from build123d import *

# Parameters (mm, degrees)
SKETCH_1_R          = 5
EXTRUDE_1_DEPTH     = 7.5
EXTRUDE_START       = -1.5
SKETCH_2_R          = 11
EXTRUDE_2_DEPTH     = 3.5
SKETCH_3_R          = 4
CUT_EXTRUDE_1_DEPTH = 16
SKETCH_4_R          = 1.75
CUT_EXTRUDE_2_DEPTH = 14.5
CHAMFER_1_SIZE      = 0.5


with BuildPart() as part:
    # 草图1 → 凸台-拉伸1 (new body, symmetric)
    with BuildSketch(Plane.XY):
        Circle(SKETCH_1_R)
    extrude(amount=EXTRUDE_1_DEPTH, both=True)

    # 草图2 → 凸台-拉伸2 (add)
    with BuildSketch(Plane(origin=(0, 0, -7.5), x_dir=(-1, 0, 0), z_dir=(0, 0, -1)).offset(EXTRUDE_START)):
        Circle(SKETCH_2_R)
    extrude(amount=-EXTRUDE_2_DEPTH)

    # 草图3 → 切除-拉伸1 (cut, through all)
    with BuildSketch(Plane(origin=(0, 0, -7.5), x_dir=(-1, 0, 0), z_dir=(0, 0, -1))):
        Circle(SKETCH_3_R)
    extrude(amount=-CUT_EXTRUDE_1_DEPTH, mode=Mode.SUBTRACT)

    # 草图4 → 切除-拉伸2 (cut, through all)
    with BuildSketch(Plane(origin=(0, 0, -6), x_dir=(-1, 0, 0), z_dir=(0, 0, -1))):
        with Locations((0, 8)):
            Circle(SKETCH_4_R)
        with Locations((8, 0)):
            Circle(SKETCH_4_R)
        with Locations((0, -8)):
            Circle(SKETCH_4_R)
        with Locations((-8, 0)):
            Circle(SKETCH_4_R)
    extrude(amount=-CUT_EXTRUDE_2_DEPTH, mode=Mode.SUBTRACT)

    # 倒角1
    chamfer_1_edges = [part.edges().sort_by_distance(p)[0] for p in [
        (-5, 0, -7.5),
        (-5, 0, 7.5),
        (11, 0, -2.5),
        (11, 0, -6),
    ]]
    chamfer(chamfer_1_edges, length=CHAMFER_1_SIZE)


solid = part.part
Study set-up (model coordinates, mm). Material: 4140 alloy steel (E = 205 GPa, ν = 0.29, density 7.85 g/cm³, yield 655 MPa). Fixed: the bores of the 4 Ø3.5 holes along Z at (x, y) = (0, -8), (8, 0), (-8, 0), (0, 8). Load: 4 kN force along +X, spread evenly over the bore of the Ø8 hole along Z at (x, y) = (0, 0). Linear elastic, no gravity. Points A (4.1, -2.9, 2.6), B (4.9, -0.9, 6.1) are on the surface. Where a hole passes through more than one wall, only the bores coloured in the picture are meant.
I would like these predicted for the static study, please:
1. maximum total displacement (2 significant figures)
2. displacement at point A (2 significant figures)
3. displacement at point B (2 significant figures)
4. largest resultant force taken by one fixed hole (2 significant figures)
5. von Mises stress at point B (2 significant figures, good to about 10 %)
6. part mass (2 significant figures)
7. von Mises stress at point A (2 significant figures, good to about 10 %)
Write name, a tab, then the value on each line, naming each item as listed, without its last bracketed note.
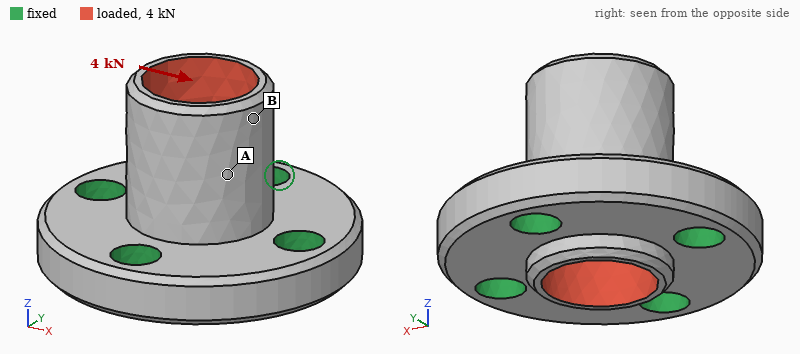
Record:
maximum total displacement	26 µm
displacement at point A	16 µm
displacement at point B	23 µm
largest resultant force taken by one fixed hole	1.7 kN
von Mises stress at point B	50 MPa
part mass	10 g
von Mises stress at point A	100 MPa
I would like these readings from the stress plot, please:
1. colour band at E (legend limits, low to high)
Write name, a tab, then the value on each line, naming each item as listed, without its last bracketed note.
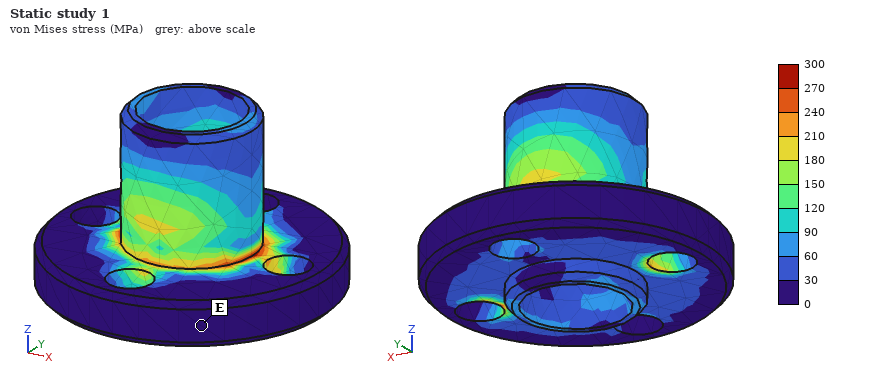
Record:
colour band at E	0 to 30 MPa
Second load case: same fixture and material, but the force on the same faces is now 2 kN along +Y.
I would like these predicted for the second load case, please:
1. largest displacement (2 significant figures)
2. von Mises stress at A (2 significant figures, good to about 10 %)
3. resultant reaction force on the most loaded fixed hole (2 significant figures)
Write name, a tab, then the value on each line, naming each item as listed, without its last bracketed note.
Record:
largest displacement	13 µm
von Mises stress at A	64 MPa
resultant reaction force on the most loaded fixed hole	840 N
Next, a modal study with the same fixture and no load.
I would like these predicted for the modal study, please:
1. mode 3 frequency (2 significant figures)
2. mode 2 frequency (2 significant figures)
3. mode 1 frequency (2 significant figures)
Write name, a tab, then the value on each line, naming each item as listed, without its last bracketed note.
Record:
mode 3 frequency	41 kHz
mode 2 frequency	41 kHz
mode 1 frequency	41 kHz
